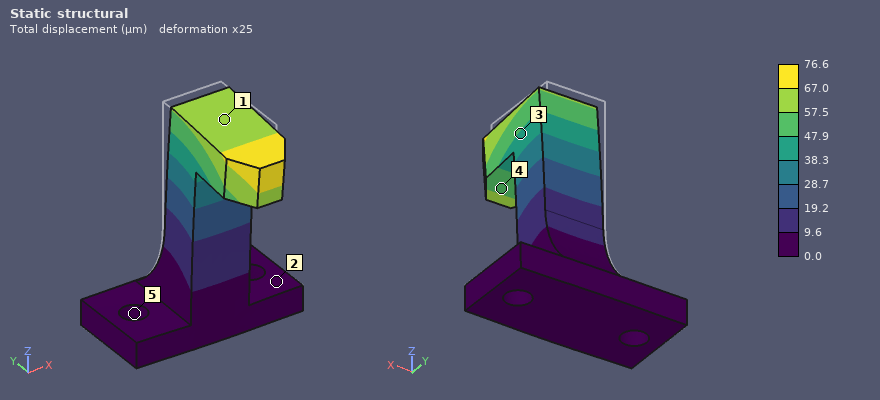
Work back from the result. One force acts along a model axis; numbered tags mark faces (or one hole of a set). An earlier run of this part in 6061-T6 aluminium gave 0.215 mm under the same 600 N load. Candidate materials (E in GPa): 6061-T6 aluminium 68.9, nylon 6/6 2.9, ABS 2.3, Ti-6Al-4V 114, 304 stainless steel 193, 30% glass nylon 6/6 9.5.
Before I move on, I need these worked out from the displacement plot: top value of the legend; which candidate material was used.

76.6 µm
304 stainless steel
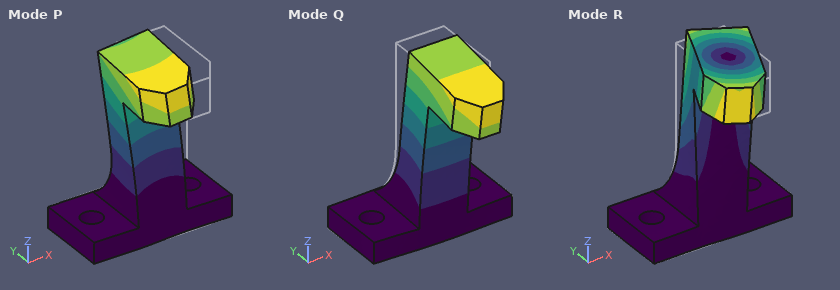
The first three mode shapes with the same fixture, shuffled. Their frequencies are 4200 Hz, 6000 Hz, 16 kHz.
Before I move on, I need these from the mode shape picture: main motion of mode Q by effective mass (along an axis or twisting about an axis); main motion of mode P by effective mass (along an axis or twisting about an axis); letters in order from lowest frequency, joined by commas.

along Y
along X
Q, P, R
